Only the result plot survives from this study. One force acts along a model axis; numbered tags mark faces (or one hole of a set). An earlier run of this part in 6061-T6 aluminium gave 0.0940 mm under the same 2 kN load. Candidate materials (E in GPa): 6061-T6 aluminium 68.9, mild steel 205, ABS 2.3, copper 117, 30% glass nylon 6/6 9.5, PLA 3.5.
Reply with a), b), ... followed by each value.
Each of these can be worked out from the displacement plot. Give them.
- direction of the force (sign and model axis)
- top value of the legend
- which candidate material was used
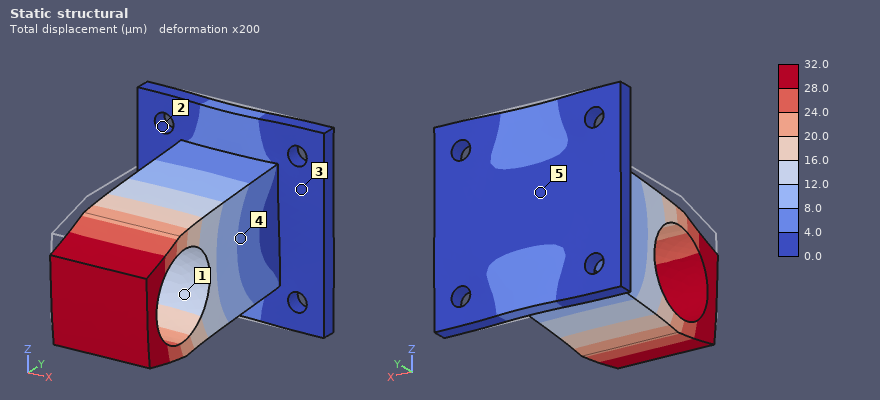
a) -Z
b) 32.0 µm
c) mild steel
